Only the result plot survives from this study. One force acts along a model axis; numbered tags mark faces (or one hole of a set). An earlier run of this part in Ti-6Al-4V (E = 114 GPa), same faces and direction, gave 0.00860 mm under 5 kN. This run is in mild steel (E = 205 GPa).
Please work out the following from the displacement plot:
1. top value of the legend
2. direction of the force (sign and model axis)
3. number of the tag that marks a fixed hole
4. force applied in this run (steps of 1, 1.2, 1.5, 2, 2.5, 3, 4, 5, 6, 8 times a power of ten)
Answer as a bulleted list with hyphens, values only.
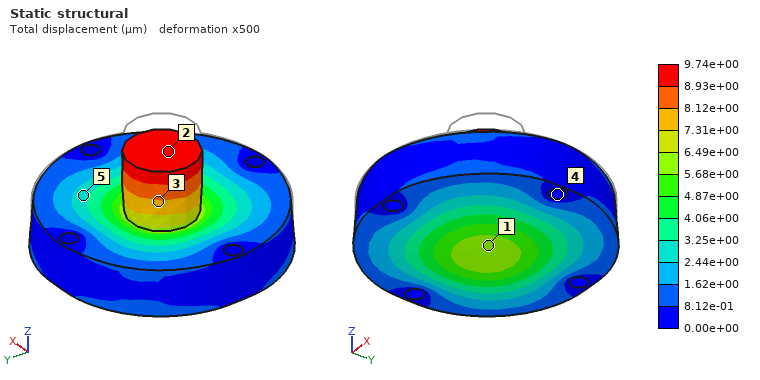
- 9.74e+00 µm
- -Z
- 4
- 10 kN
